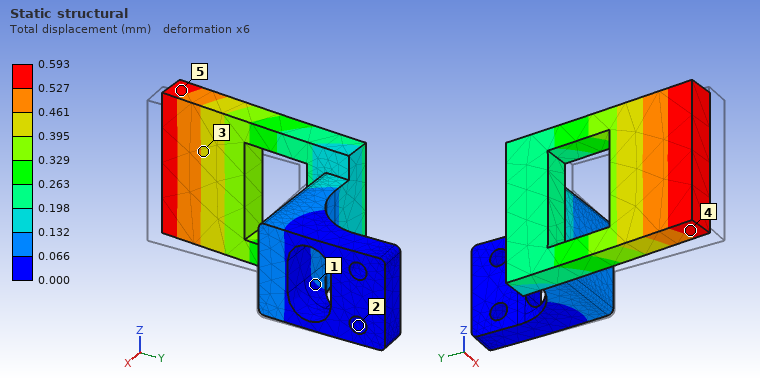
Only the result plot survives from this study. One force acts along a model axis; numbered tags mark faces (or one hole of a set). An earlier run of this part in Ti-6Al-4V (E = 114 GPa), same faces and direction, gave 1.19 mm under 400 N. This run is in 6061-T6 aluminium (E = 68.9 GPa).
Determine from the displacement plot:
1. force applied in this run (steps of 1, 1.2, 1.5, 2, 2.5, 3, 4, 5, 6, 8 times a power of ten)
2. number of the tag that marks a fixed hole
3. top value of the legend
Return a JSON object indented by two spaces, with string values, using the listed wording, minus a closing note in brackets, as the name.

{
  "force applied in this run": "120 N",
  "number of the tag that marks a fixed hole": "2",
  "top value of the legend": "0.593 mm"
}
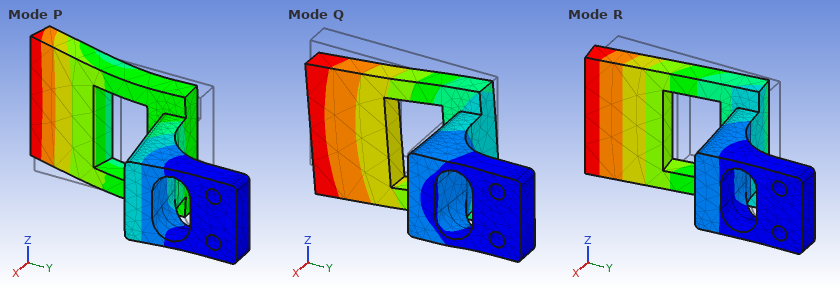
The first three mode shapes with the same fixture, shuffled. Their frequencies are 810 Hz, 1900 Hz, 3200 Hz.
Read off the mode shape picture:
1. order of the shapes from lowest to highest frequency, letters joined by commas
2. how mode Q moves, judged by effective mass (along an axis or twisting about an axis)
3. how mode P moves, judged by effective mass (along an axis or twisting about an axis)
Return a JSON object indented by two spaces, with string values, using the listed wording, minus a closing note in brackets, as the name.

{
  "order of the shapes from lowest to highest frequency, letters joined by commas": "R, Q, P",
  "how mode Q moves, judged by effective mass": "along Z",
  "how mode P moves, judged by effective mass": "along Y"
}
